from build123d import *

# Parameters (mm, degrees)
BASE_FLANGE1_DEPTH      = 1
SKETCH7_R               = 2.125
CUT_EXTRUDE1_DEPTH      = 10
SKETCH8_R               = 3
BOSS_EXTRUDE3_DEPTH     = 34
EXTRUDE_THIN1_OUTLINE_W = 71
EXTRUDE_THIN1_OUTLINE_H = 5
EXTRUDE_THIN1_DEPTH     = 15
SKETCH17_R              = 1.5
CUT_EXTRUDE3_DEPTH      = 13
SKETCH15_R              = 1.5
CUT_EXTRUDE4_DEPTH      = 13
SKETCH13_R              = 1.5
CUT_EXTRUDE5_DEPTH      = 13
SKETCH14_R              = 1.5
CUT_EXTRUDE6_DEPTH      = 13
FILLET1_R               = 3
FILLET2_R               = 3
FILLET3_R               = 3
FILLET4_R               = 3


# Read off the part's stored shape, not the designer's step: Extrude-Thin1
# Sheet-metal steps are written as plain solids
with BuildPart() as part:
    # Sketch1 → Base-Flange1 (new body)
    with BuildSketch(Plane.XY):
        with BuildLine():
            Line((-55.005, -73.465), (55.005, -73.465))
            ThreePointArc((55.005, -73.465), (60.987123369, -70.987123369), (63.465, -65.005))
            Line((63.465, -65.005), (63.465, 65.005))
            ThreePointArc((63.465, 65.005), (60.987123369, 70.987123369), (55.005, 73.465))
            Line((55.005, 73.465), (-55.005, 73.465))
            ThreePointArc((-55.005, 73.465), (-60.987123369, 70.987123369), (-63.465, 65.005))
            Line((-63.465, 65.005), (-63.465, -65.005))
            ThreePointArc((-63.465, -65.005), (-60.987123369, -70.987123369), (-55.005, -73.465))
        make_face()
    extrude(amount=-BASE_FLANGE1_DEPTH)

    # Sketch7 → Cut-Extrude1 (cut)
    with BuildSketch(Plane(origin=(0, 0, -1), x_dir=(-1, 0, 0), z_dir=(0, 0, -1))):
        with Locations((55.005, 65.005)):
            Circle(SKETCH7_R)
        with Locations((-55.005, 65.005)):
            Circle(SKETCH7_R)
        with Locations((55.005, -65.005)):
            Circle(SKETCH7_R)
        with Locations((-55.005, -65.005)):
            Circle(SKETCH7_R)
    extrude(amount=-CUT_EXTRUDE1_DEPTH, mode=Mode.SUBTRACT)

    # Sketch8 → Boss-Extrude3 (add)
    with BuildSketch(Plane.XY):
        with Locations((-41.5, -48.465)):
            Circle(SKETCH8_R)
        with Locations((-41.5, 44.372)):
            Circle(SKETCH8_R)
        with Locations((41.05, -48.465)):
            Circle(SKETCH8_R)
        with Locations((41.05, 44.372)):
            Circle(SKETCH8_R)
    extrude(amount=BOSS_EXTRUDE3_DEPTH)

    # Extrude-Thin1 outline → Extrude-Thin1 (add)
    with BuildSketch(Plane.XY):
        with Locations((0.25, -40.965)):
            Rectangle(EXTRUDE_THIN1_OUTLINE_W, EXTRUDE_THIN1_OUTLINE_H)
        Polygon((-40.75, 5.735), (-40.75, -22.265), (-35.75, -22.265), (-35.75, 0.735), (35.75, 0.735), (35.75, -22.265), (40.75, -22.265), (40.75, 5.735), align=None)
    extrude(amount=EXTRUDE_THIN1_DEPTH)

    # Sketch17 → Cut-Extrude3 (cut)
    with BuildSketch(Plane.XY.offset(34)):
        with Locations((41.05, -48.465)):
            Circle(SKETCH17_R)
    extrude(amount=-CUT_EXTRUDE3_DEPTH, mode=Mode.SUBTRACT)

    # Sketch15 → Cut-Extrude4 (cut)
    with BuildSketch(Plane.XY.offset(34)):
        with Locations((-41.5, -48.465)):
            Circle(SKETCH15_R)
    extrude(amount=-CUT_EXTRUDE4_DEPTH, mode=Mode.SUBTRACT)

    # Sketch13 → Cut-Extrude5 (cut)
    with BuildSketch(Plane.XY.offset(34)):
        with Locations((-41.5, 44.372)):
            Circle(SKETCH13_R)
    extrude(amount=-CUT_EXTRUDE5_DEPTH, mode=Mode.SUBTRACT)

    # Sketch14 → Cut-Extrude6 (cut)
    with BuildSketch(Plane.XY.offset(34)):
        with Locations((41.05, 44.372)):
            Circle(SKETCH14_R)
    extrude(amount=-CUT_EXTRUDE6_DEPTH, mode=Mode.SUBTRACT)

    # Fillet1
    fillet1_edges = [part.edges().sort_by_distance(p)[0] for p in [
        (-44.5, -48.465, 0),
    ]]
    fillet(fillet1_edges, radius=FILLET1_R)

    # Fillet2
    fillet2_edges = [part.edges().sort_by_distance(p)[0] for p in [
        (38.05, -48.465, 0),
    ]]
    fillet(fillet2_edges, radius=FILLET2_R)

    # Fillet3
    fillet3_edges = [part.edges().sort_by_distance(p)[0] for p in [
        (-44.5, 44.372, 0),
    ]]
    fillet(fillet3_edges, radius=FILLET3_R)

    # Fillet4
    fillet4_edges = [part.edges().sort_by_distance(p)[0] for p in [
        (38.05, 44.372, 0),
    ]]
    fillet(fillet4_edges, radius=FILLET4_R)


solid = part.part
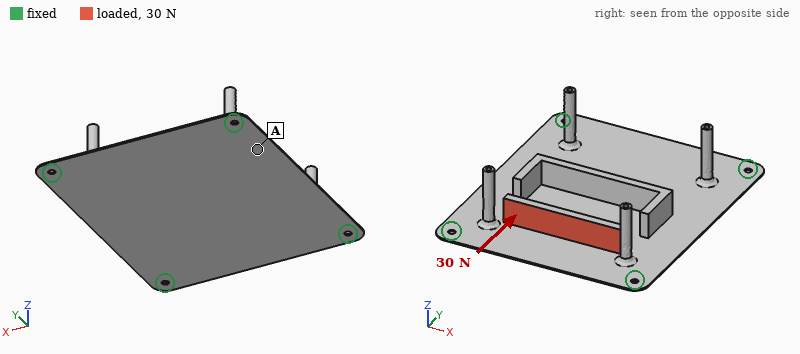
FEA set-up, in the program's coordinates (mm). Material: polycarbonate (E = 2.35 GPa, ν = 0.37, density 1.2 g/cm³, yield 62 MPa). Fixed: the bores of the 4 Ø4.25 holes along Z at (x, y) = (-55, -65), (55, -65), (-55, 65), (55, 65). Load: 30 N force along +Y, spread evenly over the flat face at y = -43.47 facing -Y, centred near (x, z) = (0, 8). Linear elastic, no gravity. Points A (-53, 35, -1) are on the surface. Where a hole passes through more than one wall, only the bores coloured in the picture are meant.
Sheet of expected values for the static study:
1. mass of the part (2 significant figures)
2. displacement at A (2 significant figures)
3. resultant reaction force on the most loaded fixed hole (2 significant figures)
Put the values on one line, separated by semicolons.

44 g; 0.91 mm; 10 N
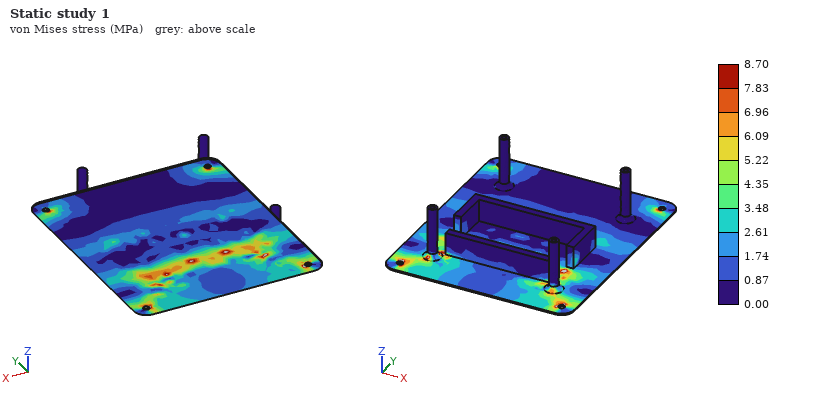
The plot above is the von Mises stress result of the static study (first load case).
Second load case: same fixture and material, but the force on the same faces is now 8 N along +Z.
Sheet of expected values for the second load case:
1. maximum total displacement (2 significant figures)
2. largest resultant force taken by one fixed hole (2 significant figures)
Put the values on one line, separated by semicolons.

2.2 mm; 4.2 N
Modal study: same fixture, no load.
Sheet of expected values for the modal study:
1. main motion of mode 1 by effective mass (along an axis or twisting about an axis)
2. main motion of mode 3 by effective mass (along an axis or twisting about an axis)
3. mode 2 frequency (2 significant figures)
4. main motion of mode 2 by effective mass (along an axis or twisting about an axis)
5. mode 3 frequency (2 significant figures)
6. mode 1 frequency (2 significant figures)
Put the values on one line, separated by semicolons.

along Z; twisting about X; 100 Hz; twisting about Y; 120 Hz; 51 Hz
